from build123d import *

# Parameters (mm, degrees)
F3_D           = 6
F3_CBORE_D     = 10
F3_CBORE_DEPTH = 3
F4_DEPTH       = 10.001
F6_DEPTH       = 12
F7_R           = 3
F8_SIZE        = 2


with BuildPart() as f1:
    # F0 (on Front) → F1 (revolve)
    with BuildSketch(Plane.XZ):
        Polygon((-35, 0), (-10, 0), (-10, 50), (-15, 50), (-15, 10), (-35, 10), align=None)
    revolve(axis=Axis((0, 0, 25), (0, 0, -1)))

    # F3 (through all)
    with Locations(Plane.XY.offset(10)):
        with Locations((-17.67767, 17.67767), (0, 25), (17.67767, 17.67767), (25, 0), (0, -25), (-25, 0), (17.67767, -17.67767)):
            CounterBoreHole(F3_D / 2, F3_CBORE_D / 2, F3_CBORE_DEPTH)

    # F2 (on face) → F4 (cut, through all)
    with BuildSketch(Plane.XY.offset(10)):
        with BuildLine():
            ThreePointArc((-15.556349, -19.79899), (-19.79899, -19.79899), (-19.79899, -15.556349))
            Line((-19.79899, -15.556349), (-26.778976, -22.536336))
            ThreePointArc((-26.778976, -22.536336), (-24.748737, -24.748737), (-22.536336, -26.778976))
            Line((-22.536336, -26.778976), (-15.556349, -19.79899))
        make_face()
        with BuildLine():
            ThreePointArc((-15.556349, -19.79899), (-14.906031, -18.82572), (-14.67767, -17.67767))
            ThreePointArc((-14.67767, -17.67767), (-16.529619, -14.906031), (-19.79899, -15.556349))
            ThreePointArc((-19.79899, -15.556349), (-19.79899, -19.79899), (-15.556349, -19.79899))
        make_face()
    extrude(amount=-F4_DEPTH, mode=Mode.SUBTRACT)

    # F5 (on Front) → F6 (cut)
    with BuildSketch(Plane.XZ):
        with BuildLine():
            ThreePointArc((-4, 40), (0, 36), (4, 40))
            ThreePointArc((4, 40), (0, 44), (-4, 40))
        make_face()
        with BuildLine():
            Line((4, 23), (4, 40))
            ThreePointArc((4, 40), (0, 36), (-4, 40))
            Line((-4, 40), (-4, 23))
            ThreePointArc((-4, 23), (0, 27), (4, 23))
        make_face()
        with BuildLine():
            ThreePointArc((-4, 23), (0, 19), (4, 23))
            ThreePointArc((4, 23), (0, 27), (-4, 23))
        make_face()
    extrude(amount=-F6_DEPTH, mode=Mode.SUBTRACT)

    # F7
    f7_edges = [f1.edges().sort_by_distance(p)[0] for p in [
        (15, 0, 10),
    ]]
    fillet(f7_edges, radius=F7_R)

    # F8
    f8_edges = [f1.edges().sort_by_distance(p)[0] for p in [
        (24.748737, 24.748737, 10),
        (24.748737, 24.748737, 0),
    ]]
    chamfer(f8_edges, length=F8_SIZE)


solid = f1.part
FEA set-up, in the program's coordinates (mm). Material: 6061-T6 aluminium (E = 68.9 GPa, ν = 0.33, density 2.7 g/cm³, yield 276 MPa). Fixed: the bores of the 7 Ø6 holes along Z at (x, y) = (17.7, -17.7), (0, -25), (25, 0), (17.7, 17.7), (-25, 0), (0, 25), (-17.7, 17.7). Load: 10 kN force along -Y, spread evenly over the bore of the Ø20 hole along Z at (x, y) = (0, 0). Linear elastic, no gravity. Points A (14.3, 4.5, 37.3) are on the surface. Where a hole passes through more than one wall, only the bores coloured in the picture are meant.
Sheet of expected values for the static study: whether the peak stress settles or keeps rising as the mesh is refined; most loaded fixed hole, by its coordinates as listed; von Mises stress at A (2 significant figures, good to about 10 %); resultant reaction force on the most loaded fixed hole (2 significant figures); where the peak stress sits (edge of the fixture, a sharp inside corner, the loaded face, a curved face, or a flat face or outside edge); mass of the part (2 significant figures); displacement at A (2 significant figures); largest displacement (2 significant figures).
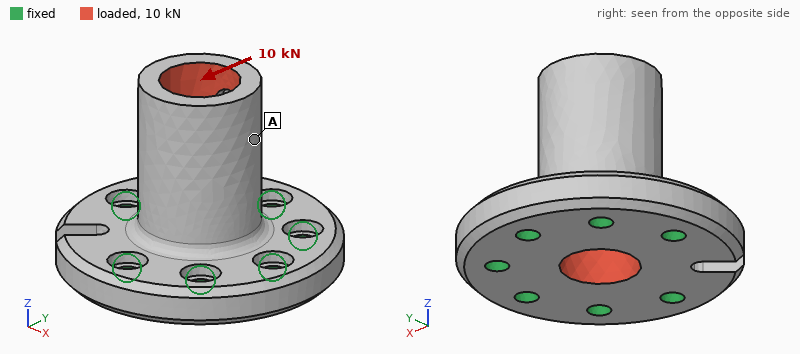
keeps rising
(0, -25)
20 MPa
4.6 kN
edge of the fixture
120 g
62 µm
94 µm
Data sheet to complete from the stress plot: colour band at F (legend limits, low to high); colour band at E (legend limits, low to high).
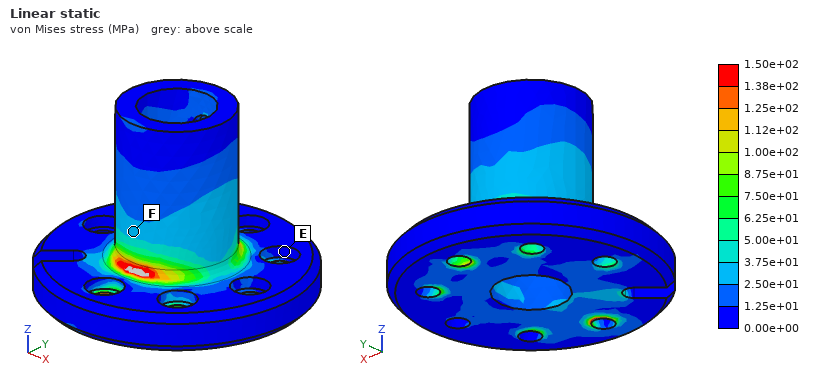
2.50e+01 to 3.75e+01 MPa
0.00e+00 to 1.25e+01 MPa
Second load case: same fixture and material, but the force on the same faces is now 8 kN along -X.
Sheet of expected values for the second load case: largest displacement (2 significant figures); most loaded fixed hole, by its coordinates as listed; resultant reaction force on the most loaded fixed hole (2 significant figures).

76 µm
(-25, 0)
3.6 kN
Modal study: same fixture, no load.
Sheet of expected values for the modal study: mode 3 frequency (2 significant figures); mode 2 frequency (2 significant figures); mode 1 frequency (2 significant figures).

18 kHz
8700 Hz
8200 Hz
